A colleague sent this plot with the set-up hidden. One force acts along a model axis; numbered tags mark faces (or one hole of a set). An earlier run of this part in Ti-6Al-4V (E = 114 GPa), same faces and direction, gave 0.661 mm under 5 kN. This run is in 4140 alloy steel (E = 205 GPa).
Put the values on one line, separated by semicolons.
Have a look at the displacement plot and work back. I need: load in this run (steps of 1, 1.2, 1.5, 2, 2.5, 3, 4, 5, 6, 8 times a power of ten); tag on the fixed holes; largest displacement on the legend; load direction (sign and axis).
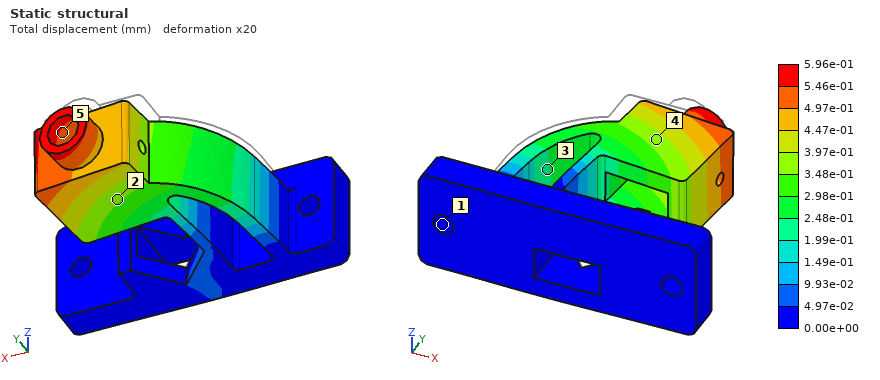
8 kN; 1; 5.96e-01 mm; +X
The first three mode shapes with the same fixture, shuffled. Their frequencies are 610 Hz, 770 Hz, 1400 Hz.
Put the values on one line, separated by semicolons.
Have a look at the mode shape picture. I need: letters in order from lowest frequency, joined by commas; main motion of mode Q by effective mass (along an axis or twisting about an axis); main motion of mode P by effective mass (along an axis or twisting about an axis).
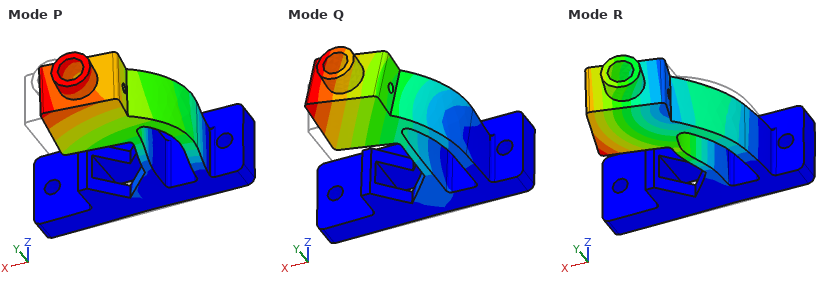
Q, P, R; along Z; along X
